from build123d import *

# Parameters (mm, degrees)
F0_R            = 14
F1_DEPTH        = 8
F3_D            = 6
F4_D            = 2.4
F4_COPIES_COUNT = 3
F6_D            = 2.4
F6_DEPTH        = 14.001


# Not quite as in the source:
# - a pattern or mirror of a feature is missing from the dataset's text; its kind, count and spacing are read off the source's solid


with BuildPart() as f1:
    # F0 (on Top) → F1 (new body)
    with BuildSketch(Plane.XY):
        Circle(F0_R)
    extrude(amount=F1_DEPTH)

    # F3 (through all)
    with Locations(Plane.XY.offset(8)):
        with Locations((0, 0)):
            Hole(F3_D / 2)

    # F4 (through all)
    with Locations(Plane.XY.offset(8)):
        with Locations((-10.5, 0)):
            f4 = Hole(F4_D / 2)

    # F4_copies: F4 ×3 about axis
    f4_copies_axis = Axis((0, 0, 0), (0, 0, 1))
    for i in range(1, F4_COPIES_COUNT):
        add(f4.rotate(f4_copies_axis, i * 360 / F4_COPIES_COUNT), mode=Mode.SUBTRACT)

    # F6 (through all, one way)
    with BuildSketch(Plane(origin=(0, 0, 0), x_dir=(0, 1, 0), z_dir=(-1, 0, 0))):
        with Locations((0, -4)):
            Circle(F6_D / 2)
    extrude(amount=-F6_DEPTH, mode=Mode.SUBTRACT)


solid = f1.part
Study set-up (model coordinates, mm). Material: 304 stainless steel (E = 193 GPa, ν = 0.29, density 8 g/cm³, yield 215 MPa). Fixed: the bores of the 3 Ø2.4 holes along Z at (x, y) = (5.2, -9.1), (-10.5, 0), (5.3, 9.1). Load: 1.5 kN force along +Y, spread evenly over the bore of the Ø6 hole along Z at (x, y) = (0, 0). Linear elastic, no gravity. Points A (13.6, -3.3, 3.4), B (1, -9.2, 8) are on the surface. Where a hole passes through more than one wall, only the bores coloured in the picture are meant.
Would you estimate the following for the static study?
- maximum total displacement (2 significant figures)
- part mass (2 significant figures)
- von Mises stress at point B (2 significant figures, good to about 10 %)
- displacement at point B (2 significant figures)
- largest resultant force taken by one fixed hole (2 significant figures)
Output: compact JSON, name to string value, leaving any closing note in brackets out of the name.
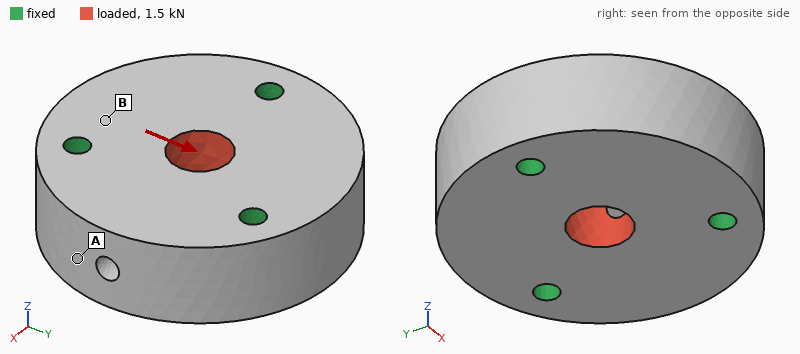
{"maximum total displacement": "0.62 µm", "part mass": "36 g", "von Mises stress at point B": "6.3 MPa", "displacement at point B": "0.27 µm", "largest resultant force taken by one fixed hole": "500 N"}
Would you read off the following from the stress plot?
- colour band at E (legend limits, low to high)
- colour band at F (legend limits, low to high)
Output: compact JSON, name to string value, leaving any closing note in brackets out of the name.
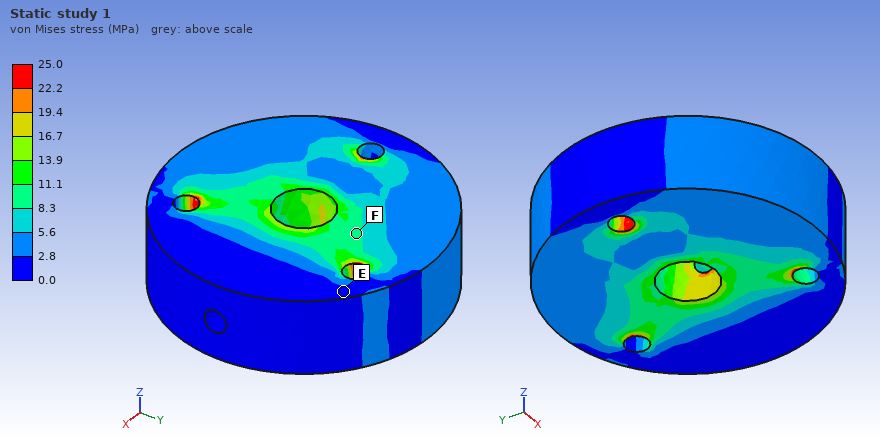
{"colour band at E": "0.0 to 2.8 MPa", "colour band at F": "8.3 to 11.1 MPa"}
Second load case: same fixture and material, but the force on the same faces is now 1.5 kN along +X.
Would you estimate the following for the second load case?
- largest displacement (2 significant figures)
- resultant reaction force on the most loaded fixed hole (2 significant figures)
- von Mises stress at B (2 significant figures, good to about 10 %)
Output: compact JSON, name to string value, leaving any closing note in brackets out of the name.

{"largest displacement": "0.64 µm", "resultant reaction force on the most loaded fixed hole": "530 N", "von Mises stress at B": "4.5 MPa"}
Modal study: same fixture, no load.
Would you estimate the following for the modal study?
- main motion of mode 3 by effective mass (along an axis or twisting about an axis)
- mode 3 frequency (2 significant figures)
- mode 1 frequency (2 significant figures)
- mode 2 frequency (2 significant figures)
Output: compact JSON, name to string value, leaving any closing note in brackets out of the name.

{"main motion of mode 3 by effective mass": "along Z", "mode 3 frequency": "51 kHz", "mode 1 frequency": "46 kHz", "mode 2 frequency": "46 kHz"}
